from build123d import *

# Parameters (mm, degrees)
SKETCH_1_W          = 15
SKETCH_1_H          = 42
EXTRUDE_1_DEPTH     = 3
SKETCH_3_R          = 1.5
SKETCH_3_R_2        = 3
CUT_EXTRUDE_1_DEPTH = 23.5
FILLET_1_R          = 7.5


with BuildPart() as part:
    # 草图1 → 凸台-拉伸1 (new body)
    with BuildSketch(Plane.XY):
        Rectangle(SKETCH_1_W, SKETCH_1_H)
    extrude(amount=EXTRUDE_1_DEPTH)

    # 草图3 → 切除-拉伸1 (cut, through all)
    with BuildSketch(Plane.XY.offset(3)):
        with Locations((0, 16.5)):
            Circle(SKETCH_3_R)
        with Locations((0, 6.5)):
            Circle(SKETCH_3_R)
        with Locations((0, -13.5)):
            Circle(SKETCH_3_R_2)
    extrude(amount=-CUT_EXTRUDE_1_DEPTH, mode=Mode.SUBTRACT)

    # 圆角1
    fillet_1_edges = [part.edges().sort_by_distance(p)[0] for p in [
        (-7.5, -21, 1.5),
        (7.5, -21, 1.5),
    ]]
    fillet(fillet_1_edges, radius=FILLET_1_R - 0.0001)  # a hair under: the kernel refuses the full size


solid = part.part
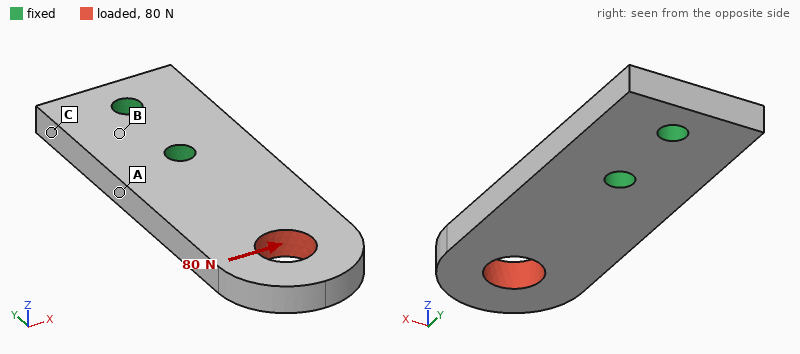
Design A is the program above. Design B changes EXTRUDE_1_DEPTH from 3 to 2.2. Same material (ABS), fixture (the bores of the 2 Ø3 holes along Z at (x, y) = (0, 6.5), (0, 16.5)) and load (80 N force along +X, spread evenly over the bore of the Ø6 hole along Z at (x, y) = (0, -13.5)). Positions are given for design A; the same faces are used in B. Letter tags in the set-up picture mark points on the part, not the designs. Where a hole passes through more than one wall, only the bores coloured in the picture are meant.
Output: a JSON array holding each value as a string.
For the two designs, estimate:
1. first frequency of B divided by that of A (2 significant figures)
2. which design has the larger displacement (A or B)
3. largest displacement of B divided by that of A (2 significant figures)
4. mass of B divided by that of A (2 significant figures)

["0.75", "B", "1.4", "0.73"]
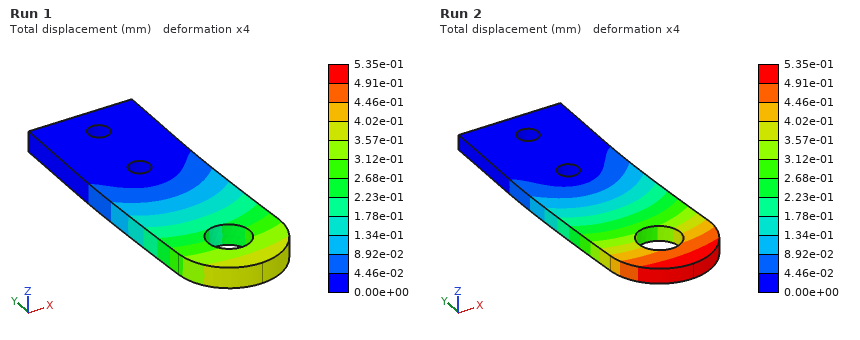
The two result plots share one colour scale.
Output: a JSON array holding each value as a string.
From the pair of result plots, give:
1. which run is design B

["Run 2"]
